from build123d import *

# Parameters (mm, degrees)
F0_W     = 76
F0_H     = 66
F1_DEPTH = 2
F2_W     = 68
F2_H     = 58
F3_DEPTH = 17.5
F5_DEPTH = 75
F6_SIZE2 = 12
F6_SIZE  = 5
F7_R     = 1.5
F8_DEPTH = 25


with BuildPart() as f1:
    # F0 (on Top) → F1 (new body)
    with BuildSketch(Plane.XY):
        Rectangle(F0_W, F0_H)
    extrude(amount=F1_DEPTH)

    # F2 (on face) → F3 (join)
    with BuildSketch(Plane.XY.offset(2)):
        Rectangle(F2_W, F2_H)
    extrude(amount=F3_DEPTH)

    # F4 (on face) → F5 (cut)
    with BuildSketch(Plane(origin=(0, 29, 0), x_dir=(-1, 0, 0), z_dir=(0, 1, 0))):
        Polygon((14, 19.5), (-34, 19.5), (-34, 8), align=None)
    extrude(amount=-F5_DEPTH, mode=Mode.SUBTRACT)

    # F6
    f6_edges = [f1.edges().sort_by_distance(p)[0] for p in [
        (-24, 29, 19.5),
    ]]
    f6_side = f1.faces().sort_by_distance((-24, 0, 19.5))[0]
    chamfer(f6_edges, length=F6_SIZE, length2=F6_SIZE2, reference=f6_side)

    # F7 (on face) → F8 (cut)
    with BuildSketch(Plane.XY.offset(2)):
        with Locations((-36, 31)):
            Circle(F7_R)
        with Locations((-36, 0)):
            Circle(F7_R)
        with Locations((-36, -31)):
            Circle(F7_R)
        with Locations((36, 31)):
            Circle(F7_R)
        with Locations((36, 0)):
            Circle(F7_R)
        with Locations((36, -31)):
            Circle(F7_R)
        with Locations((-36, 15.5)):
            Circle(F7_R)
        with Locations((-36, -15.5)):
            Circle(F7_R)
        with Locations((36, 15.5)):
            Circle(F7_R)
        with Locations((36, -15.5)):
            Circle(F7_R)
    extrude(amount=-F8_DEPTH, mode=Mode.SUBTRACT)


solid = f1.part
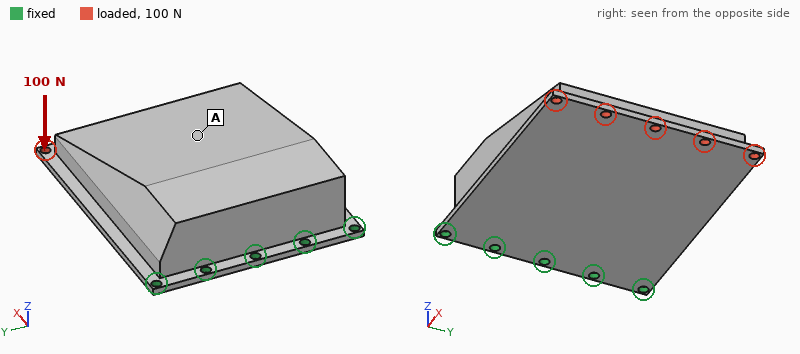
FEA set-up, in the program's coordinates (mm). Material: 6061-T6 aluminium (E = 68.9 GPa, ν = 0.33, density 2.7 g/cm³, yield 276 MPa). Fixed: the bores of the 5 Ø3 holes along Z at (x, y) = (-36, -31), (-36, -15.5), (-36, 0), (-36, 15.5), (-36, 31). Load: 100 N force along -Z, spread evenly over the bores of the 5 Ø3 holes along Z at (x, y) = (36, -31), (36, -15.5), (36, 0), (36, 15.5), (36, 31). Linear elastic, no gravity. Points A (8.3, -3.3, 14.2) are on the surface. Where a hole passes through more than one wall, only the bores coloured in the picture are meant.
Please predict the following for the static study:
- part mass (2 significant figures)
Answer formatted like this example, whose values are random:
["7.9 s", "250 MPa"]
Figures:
["170 g"]
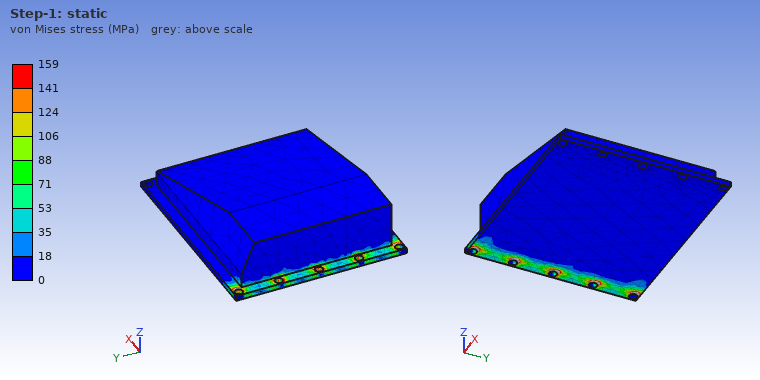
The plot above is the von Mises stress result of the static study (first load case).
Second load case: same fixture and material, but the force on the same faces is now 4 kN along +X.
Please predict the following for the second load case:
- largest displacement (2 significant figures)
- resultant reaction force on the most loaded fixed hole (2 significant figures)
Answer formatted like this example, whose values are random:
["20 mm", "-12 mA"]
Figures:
["97 µm", "970 N"]
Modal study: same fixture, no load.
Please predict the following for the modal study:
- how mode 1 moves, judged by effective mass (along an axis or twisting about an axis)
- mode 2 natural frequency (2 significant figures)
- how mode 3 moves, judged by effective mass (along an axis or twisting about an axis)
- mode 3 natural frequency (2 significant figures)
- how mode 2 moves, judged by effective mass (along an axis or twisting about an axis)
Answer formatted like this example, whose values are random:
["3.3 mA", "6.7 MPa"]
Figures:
["along Z", "4100 Hz", "along Y", "5200 Hz", "along Y"]
